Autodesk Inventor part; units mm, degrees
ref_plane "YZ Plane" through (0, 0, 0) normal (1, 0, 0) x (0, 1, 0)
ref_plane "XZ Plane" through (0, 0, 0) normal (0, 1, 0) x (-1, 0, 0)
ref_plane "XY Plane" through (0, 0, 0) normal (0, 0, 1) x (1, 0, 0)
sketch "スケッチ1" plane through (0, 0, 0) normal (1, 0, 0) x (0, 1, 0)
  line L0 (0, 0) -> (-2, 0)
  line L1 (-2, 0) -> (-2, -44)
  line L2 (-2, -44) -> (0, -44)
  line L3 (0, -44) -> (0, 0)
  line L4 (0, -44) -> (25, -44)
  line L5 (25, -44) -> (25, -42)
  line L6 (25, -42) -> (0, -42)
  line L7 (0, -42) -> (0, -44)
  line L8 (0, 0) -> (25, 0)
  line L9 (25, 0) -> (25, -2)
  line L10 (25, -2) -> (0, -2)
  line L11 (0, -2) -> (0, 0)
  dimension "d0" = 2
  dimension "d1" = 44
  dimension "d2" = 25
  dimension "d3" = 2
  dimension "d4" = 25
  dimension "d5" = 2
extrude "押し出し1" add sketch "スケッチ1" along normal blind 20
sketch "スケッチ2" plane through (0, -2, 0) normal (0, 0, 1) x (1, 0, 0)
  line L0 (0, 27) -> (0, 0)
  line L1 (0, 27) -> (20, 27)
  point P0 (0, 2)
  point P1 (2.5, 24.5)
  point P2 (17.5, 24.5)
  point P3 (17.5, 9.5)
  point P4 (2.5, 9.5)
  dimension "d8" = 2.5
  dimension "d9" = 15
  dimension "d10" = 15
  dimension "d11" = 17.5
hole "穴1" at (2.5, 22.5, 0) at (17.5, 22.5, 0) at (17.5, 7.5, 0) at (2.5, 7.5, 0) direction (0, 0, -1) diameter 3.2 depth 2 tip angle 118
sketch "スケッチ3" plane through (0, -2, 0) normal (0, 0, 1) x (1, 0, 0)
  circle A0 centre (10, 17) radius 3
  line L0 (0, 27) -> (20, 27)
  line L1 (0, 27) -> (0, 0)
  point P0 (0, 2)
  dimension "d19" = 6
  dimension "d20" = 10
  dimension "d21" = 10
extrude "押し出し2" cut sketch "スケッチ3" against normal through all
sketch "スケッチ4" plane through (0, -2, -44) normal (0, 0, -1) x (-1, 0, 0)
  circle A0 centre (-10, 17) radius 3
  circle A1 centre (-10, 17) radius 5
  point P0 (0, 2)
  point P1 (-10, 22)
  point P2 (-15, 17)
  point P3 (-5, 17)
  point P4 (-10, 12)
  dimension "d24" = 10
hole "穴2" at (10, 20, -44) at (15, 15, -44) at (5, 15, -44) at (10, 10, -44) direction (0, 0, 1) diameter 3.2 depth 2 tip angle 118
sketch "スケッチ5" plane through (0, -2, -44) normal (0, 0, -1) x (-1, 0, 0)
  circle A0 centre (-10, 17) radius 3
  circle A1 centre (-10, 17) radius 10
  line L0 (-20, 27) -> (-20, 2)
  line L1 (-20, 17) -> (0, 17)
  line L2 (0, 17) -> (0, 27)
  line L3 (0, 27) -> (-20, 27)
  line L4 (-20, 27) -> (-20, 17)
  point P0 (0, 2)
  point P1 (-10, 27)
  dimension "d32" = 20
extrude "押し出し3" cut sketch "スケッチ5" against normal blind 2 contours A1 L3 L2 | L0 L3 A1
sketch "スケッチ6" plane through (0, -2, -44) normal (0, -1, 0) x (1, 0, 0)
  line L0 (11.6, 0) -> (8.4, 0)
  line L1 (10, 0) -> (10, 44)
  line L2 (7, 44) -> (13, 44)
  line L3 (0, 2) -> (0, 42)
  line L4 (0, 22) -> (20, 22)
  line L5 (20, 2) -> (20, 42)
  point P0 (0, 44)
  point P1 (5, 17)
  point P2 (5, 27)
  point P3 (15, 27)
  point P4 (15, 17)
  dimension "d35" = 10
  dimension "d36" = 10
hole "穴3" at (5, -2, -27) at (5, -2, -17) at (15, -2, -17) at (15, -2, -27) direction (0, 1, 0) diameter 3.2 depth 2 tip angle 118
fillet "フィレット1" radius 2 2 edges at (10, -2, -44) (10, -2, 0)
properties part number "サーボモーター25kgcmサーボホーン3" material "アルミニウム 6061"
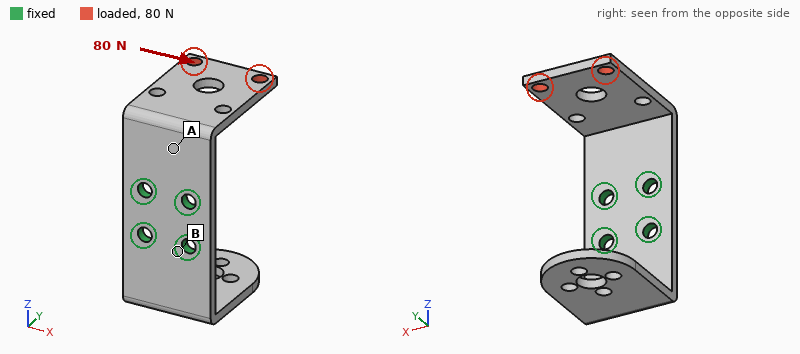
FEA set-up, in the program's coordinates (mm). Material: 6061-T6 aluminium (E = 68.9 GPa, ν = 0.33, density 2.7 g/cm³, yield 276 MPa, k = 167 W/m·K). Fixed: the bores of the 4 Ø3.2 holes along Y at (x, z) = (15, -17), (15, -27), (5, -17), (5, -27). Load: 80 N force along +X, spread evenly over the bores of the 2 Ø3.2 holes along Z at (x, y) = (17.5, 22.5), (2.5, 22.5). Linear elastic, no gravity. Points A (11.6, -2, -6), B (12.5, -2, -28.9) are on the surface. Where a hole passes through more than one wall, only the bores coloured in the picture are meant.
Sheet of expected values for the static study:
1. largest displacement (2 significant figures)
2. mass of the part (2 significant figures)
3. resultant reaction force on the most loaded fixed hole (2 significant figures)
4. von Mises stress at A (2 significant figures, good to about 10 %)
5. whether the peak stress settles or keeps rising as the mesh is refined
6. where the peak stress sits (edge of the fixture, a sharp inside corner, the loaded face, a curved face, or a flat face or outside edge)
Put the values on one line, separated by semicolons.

0.37 mm; 9.0 g; 180 N; 88 MPa; keeps rising; edge of the fixture
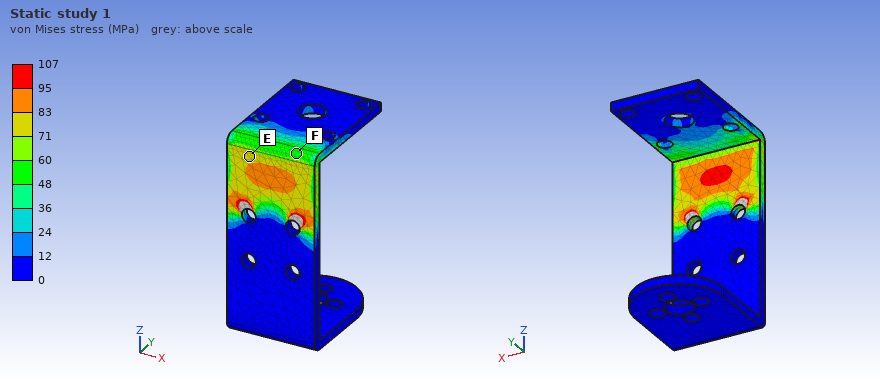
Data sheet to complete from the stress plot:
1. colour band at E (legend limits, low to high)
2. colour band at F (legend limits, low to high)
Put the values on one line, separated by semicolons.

71 to 83 MPa; 48 to 60 MPa
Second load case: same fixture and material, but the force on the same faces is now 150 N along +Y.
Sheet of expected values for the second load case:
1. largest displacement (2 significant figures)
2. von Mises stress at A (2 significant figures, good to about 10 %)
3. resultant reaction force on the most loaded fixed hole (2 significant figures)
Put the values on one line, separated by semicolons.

0.51 mm; 50 MPa; 86 N
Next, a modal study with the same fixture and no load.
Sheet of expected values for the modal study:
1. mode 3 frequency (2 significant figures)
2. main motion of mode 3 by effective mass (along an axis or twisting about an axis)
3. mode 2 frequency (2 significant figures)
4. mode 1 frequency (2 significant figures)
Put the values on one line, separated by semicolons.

2400 Hz; along X; 1500 Hz; 1300 Hz
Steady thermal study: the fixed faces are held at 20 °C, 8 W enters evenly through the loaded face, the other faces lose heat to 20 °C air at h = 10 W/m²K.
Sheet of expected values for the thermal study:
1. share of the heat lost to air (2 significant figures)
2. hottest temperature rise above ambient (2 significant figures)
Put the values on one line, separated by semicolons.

5.7 %; 56 K
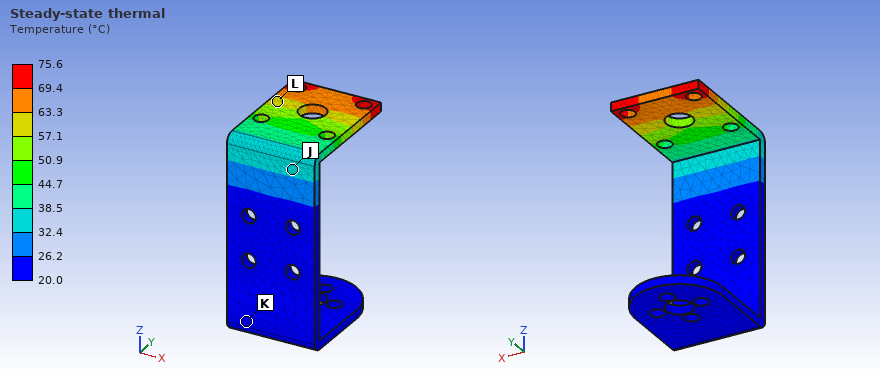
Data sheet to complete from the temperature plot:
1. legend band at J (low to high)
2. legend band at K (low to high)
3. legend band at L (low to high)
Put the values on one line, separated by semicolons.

32.4 to 38.5 °C; 20.0 to 26.2 °C; 57.1 to 63.3 °C
